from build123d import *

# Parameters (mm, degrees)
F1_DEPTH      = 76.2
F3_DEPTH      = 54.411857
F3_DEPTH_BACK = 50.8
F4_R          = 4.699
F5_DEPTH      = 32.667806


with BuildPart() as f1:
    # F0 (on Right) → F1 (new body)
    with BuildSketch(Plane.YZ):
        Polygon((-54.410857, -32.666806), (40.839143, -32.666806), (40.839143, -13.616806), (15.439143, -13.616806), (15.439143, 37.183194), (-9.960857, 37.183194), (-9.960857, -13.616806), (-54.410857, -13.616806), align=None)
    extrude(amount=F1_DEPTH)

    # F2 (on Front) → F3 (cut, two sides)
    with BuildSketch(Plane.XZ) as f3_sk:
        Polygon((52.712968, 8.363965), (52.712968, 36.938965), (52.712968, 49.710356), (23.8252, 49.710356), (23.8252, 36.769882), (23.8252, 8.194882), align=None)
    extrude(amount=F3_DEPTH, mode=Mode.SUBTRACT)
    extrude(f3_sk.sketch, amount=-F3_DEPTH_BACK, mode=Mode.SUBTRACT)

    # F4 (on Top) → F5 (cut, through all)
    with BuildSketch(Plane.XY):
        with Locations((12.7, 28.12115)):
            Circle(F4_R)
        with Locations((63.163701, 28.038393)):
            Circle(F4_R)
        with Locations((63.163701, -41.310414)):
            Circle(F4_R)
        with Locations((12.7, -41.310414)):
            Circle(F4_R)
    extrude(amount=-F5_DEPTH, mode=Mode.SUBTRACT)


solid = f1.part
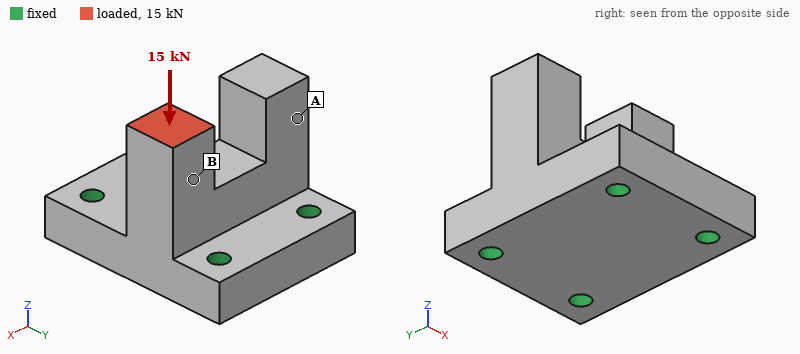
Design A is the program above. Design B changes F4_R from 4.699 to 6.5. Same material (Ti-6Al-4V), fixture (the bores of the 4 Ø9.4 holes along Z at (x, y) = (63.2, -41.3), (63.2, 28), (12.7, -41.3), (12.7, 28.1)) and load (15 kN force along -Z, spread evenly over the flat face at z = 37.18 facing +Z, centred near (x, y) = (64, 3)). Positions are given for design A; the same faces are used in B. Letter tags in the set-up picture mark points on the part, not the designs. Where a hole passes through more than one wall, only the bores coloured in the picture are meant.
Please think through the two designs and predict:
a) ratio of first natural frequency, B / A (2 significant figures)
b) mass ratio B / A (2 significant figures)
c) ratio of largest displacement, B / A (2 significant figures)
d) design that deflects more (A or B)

1.0
0.98
0.91
A
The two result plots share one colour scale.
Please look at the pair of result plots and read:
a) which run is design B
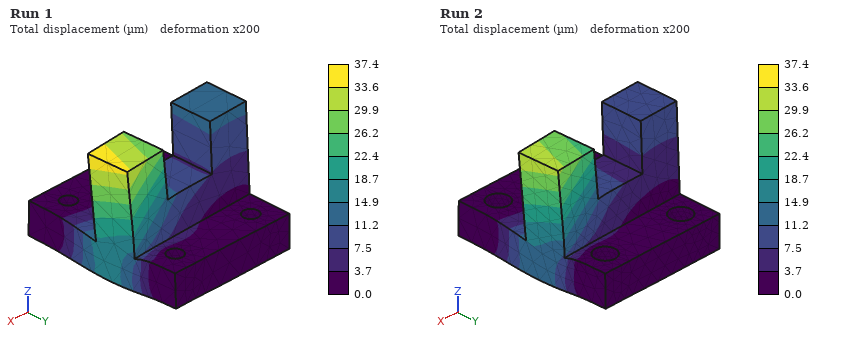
Run 2
